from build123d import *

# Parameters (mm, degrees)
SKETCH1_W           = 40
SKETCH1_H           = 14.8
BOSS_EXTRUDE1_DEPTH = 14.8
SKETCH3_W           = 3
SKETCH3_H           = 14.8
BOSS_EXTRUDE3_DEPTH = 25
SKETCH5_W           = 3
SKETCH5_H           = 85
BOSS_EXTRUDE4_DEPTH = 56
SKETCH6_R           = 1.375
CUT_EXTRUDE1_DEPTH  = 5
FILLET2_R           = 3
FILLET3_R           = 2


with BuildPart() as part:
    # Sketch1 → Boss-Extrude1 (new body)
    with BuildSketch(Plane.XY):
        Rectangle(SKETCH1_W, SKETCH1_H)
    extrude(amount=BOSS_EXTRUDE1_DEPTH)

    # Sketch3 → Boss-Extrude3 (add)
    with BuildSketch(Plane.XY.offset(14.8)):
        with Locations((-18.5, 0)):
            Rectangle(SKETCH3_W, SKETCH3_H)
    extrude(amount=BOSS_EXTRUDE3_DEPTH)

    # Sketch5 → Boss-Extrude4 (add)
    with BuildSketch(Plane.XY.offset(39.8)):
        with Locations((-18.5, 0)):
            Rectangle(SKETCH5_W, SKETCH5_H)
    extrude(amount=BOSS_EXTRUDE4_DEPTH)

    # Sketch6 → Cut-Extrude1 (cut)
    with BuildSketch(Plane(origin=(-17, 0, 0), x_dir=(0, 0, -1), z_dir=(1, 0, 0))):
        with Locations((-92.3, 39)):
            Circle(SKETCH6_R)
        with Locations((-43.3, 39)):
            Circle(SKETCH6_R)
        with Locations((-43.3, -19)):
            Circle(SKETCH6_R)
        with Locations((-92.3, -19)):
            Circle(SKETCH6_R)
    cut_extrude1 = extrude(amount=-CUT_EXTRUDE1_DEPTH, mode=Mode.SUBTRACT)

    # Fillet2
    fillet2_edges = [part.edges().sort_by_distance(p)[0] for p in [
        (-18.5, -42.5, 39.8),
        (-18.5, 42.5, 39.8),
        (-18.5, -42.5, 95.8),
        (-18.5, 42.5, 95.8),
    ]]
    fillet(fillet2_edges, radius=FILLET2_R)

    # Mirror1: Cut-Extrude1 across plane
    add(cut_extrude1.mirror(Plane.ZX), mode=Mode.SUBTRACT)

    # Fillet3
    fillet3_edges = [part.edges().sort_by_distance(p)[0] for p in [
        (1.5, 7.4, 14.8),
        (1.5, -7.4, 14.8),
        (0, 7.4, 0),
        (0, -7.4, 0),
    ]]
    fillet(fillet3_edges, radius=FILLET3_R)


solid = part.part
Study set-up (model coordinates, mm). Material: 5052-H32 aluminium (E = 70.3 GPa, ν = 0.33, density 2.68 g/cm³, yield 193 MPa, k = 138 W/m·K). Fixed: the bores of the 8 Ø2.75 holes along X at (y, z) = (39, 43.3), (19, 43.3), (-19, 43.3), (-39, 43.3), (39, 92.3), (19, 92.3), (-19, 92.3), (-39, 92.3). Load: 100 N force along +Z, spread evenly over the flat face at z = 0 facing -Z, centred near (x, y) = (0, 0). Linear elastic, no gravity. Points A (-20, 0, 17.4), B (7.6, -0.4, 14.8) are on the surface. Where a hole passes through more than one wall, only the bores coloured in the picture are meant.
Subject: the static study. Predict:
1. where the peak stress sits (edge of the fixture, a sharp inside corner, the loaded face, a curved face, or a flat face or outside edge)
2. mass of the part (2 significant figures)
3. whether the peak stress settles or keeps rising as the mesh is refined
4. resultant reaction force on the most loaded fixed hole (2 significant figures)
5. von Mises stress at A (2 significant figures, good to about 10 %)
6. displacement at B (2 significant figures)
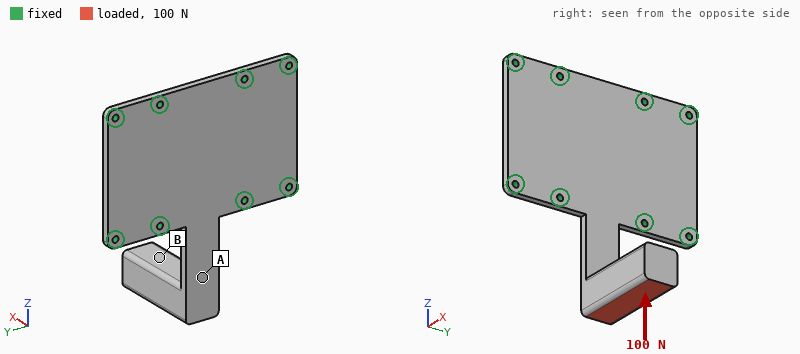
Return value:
a sharp inside corner
64 g
keeps rising
31 N
73 MPa
0.80 mm
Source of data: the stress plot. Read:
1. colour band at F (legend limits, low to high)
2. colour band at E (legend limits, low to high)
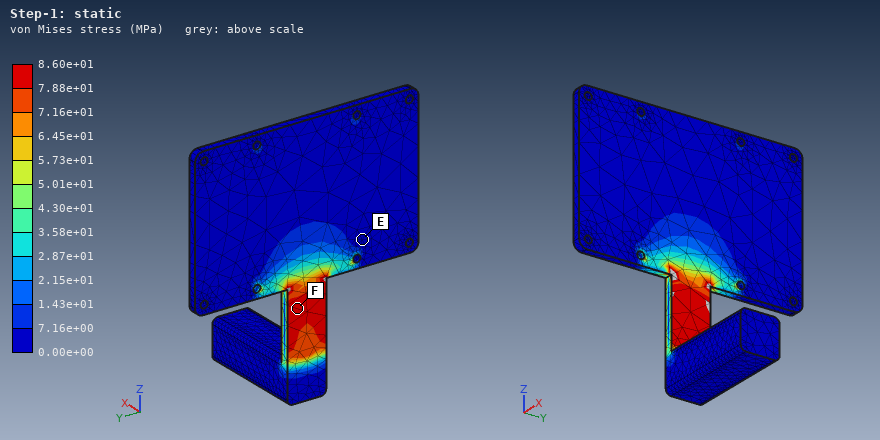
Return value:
7.88e+01 to 8.60e+01 MPa
0.00e+00 to 7.16e+00 MPa
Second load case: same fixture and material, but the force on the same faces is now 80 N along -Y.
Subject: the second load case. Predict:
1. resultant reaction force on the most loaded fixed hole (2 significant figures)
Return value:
97 N
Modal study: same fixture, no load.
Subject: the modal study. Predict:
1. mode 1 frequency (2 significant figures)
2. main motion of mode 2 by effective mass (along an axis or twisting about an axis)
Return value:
270 Hz
along Y
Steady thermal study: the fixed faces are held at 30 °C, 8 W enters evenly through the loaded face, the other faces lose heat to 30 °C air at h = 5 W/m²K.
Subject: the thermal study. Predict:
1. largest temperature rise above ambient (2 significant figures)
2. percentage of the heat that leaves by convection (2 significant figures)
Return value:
50 K
8.9 %
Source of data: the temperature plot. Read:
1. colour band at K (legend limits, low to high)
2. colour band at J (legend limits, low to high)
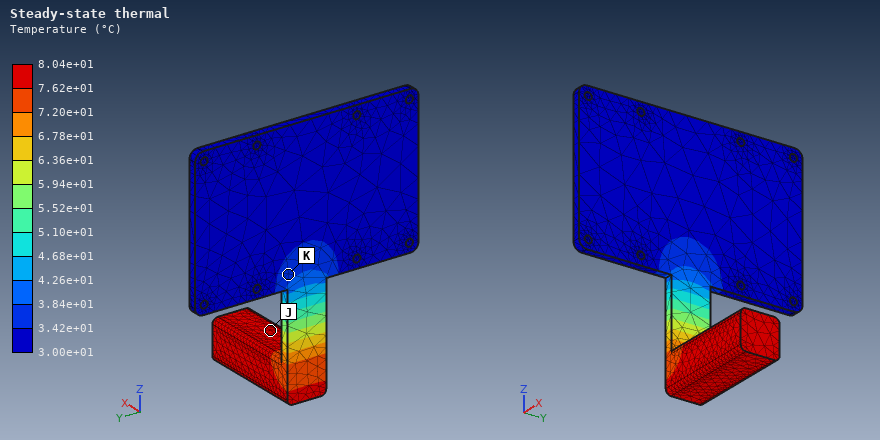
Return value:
3.42e+01 to 3.84e+01 °C
7.62e+01 to 8.04e+01 °C
